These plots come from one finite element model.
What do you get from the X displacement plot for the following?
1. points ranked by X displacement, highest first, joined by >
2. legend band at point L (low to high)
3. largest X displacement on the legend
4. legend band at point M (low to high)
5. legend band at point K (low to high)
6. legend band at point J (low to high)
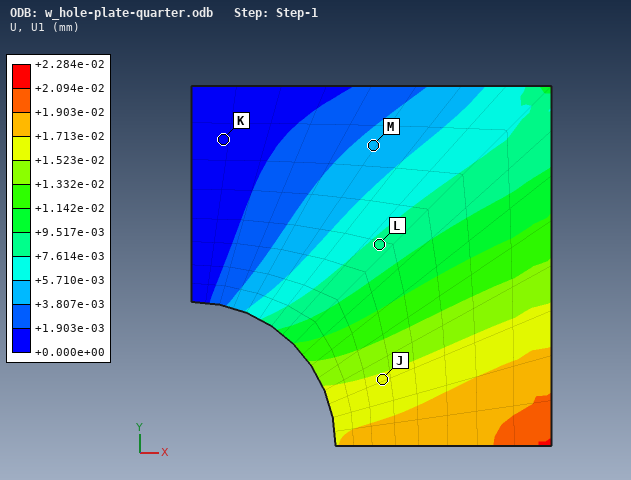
J > L > M > K
+7.614e-03 to +9.517e-03 mm
+2.284e-02 mm
+3.807e-03 to +5.710e-03 mm
+0.000e+00 to +1.903e-03 mm
+1.523e-02 to +1.713e-02 mm
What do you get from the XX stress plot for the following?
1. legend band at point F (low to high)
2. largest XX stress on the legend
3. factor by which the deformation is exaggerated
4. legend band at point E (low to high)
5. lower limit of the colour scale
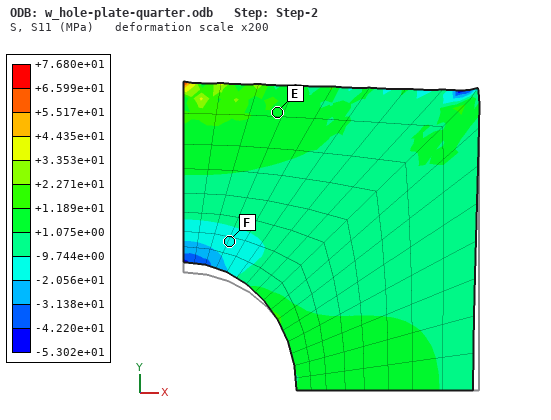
-2.056e+01 to -9.744e+00 MPa
+7.680e+01 MPa
200
+1.075e+00 to +1.189e+01 MPa
-5.302e+01 MPa
